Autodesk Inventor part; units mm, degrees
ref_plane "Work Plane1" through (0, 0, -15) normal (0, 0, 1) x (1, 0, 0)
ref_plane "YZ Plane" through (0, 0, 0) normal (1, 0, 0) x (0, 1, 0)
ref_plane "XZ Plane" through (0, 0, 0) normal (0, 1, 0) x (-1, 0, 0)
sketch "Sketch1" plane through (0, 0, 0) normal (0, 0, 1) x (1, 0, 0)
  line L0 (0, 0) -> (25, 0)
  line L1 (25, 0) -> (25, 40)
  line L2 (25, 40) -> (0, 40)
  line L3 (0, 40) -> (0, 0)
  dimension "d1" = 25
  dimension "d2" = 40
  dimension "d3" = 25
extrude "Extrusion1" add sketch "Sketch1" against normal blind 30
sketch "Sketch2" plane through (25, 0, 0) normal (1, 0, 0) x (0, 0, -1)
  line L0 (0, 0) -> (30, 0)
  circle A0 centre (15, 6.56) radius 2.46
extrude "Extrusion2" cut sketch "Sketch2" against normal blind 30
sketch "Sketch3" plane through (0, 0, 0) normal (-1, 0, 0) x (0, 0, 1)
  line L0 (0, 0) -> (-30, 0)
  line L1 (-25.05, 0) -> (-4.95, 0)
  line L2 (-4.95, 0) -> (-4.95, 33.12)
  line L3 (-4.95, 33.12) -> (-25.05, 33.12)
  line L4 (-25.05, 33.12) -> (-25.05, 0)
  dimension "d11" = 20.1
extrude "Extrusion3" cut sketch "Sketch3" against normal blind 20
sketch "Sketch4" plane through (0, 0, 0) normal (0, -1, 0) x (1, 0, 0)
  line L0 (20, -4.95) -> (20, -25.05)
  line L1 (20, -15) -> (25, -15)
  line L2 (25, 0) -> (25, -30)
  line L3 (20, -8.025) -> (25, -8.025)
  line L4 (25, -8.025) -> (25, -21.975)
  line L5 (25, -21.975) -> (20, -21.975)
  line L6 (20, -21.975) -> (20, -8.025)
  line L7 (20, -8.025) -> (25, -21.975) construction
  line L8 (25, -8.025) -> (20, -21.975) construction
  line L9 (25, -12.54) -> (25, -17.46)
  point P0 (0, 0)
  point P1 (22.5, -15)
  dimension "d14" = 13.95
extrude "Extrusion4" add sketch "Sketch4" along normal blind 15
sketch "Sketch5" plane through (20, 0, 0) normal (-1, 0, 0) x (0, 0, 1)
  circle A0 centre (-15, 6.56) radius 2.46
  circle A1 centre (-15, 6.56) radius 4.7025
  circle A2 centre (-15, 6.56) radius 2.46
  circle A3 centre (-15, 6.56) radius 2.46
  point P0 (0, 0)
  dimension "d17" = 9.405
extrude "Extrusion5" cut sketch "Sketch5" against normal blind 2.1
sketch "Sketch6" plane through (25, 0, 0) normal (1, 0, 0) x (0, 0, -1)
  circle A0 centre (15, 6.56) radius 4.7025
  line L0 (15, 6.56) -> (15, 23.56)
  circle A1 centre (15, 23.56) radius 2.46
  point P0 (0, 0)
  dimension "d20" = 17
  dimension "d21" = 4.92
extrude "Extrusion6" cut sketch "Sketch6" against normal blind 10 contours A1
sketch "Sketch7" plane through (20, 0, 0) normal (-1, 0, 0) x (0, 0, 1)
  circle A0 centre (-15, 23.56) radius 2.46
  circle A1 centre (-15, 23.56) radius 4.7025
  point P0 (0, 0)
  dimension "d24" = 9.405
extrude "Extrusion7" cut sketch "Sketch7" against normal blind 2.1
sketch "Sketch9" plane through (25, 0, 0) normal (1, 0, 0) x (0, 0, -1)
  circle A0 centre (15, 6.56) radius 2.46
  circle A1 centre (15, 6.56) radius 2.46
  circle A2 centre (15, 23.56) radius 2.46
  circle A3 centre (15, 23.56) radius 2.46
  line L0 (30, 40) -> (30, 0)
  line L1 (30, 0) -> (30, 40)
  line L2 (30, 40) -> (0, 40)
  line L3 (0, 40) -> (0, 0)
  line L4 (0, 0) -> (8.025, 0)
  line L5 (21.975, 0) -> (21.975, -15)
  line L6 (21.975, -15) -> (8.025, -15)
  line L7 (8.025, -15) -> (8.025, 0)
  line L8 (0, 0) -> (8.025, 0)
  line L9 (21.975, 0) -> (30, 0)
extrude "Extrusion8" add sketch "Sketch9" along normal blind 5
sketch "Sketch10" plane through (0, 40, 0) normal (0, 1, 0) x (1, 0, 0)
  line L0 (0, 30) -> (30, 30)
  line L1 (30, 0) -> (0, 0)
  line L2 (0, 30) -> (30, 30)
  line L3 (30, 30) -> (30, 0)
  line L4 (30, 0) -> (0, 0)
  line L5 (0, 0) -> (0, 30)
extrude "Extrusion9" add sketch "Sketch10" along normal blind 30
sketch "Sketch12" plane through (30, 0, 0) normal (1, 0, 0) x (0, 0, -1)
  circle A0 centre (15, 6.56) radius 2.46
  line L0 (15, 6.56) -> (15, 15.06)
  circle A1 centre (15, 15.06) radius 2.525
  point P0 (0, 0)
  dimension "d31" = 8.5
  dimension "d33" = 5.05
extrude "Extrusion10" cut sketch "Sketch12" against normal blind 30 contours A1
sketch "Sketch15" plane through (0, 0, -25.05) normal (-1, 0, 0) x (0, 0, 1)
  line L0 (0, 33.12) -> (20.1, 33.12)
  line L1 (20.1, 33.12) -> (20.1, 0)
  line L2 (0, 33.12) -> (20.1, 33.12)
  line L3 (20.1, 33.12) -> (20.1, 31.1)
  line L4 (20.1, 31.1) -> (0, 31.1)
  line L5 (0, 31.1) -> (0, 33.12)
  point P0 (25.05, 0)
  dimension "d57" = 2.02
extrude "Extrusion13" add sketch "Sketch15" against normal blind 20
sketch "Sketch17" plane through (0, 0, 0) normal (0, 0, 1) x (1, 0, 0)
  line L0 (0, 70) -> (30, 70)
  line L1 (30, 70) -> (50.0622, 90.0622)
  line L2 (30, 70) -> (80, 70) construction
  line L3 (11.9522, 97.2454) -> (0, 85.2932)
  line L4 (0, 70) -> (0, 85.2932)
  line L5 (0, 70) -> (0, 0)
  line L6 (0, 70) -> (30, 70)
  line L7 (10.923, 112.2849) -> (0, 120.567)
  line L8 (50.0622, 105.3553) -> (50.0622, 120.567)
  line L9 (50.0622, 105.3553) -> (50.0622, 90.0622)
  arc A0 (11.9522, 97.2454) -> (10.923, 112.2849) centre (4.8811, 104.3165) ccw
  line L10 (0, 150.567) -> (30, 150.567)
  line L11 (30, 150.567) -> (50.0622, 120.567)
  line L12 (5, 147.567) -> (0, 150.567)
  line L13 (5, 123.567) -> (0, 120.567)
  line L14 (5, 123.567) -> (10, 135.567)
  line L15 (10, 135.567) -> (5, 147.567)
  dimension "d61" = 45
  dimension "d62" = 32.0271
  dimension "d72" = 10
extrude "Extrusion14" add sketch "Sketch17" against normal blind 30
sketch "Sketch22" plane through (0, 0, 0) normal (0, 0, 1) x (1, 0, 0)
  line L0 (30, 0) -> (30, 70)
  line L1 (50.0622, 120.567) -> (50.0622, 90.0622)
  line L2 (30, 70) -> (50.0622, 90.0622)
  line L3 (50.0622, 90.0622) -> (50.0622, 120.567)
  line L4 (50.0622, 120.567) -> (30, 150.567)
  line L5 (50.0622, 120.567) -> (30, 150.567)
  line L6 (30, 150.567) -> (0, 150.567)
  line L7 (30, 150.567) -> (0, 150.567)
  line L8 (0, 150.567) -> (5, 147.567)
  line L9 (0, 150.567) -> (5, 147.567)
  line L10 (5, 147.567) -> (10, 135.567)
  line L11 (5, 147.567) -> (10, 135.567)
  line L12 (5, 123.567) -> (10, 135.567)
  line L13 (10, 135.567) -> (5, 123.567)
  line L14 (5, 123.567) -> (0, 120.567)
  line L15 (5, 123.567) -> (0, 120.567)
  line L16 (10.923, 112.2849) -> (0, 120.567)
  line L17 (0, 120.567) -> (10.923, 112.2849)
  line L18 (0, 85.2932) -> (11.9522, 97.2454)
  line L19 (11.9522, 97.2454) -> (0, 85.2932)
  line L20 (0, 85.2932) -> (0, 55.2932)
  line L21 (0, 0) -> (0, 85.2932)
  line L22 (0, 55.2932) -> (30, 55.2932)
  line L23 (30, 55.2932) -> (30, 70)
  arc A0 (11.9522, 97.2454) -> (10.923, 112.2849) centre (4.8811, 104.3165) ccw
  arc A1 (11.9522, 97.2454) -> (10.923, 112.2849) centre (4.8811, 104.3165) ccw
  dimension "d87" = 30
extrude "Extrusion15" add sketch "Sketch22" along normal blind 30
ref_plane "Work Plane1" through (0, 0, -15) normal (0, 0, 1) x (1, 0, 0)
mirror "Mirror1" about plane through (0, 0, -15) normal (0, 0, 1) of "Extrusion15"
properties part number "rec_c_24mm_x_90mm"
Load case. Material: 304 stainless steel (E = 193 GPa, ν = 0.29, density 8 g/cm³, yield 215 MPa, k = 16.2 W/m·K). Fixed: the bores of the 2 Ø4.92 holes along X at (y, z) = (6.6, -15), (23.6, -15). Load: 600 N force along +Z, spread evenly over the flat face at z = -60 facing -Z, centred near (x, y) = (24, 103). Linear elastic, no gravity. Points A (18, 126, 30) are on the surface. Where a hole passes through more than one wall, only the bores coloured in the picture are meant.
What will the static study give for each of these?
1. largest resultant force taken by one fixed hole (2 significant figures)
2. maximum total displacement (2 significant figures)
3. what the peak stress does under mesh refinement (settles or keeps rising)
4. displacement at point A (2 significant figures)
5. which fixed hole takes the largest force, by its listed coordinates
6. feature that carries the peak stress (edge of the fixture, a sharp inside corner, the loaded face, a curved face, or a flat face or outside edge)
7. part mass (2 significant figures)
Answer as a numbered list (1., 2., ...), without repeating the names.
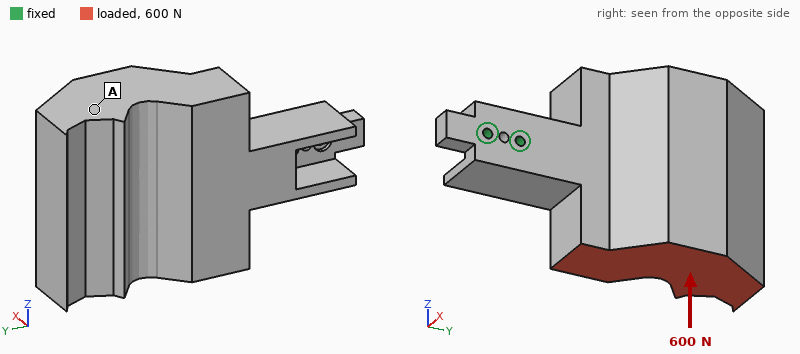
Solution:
1. 2.6 kN
2. 46 µm
3. keeps rising
4. 38 µm
5. (23.6, -15)
6. edge of the fixture
7. 2.8 kg
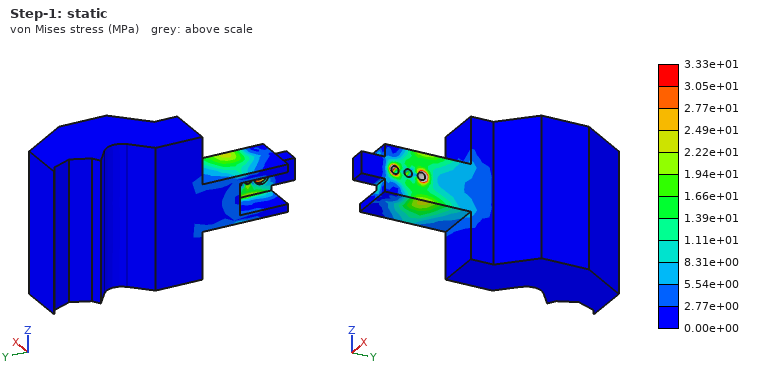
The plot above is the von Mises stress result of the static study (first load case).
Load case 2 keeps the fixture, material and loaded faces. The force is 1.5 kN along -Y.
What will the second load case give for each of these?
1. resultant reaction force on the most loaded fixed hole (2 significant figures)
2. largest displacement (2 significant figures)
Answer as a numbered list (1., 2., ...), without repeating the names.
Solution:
1. 3.1 kN
2. 73 µm
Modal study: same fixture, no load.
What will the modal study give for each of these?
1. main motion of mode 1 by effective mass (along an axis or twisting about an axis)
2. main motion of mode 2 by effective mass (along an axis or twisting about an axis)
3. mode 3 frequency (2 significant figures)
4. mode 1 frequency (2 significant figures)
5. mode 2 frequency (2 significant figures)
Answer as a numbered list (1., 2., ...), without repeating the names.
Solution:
1. along X
2. along Z
3. 780 Hz
4. 390 Hz
5. 430 Hz
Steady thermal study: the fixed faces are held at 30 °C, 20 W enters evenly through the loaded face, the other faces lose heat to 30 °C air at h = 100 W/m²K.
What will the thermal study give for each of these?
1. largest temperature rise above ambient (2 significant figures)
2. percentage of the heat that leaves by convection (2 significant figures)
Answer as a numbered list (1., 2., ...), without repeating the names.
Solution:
1. 17 K
2. 97 %
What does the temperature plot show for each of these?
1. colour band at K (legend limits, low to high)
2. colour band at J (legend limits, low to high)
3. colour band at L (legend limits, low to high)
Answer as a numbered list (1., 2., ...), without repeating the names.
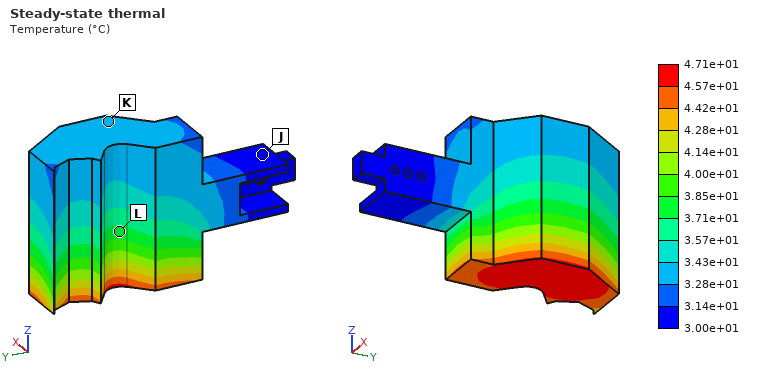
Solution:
1. 3.28e+01 to 3.43e+01 °C
2. 3.00e+01 to 3.14e+01 °C
3. 3.71e+01 to 3.85e+01 °C
